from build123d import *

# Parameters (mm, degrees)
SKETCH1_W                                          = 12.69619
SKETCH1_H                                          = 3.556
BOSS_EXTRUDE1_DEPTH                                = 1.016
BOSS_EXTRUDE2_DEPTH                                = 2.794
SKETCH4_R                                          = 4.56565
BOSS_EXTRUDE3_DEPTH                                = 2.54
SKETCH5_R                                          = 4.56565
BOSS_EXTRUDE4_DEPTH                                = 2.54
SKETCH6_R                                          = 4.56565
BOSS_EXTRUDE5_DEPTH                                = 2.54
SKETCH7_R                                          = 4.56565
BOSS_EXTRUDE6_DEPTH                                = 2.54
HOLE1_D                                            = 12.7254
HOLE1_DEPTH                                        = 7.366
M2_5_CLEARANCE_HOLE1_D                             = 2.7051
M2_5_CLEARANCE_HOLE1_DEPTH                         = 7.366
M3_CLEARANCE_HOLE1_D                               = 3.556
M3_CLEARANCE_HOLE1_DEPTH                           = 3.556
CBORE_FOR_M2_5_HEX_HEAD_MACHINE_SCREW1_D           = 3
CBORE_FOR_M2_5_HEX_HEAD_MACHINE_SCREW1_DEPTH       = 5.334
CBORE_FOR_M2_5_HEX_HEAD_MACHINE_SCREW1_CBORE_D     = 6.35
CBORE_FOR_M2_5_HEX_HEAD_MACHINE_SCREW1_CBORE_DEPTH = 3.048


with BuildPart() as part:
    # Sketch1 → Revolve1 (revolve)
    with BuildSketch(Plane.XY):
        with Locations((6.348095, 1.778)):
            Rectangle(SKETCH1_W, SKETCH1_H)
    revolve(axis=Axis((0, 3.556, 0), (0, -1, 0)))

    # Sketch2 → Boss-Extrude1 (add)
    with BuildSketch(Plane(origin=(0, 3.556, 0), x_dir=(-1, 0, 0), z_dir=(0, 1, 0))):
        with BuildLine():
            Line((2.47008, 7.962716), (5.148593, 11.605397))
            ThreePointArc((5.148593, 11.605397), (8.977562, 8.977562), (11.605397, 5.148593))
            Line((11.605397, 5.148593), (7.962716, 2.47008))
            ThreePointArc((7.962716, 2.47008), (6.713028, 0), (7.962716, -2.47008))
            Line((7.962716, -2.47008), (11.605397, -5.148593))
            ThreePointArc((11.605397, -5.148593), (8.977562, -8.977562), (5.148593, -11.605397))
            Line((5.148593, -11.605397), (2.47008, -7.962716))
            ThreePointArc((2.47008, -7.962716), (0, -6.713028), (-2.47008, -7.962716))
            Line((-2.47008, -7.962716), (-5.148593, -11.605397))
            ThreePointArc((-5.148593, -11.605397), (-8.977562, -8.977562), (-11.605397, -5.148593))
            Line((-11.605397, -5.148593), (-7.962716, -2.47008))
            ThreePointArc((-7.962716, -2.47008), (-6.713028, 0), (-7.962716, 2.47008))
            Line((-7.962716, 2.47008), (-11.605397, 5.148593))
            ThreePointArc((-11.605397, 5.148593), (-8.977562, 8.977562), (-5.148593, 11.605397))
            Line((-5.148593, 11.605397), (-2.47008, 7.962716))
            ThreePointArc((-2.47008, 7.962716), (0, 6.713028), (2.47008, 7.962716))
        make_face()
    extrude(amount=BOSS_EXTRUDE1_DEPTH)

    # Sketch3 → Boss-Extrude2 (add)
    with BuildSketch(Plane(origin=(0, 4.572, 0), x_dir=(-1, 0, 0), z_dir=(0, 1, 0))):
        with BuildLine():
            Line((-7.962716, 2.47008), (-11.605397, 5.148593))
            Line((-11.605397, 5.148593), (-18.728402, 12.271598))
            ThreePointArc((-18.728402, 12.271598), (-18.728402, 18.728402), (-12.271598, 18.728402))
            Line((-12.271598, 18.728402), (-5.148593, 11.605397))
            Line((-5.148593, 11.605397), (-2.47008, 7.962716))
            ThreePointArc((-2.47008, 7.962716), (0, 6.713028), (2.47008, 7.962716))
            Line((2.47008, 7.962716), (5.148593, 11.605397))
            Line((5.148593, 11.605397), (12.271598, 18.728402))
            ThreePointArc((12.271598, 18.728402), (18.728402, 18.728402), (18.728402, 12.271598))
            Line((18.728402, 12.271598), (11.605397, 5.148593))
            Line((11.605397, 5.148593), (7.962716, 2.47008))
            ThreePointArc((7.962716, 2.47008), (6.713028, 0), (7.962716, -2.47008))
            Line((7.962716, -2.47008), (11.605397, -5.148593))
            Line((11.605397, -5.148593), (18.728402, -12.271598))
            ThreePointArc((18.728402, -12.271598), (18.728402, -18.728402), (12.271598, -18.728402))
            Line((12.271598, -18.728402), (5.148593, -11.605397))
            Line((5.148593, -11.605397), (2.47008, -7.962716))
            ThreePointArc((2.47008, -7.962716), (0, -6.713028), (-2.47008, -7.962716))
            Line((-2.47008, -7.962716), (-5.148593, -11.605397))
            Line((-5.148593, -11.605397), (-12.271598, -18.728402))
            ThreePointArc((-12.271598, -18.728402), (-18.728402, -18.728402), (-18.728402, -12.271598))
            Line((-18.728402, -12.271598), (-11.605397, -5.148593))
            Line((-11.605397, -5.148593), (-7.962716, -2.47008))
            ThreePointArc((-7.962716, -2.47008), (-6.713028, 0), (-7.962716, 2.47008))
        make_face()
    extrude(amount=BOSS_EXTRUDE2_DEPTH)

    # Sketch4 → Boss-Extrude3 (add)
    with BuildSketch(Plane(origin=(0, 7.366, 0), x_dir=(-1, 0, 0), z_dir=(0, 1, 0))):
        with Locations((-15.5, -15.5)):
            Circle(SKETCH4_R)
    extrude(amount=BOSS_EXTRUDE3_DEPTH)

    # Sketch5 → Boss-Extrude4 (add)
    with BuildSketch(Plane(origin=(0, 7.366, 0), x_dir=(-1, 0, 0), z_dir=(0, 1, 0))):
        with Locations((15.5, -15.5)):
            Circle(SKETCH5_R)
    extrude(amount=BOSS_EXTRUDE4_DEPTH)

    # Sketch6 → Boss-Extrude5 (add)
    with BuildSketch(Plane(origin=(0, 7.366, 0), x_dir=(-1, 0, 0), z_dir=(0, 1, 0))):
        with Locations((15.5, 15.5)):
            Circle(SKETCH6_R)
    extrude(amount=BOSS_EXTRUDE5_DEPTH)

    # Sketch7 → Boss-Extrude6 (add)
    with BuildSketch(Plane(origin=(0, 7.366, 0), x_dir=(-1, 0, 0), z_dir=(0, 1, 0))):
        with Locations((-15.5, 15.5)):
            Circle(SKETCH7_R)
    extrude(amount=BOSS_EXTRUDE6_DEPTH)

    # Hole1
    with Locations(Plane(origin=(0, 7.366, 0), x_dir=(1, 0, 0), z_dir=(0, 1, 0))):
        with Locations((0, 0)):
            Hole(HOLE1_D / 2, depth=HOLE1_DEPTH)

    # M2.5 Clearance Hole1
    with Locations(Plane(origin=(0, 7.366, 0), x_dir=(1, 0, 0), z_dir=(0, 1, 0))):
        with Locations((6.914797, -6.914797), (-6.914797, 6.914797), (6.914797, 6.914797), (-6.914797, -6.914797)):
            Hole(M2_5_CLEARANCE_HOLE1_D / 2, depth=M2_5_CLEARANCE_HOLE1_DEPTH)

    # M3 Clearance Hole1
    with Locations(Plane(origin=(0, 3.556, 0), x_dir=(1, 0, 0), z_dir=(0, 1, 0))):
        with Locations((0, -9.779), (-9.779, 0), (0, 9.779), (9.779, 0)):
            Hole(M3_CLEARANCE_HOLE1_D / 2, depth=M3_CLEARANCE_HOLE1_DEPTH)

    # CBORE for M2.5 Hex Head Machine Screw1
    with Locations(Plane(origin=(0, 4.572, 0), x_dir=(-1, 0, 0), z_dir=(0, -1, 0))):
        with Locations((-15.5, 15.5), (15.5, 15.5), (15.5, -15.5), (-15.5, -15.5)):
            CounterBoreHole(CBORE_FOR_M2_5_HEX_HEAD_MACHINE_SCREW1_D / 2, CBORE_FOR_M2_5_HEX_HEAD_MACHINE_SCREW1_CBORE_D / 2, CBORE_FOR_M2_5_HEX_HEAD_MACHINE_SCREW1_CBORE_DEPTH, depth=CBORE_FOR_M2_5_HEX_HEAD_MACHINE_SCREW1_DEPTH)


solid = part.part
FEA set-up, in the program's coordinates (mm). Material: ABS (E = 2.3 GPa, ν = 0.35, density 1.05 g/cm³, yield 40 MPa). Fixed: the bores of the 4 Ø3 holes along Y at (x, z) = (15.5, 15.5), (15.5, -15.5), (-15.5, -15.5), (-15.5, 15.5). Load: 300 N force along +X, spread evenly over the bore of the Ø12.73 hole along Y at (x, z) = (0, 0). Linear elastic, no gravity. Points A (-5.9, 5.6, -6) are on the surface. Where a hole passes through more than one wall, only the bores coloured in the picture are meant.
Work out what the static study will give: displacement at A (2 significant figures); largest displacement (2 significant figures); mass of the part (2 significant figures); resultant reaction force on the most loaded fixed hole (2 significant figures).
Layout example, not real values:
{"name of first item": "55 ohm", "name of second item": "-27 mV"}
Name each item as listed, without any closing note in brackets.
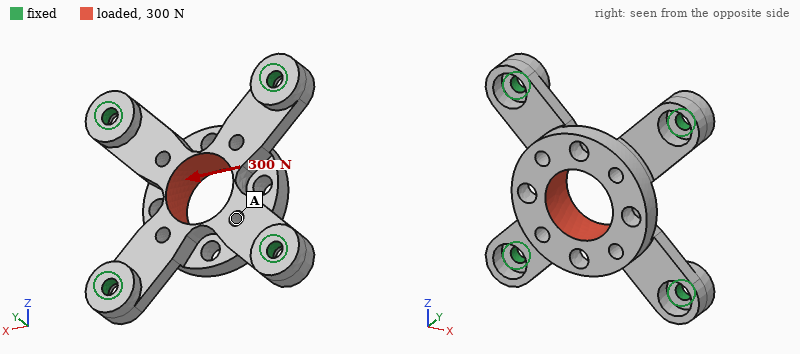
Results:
{"displacement at A": "72 µm", "largest displacement": "98 µm", "mass of the part": "3.6 g", "resultant reaction force on the most loaded fixed hole": "91 N"}
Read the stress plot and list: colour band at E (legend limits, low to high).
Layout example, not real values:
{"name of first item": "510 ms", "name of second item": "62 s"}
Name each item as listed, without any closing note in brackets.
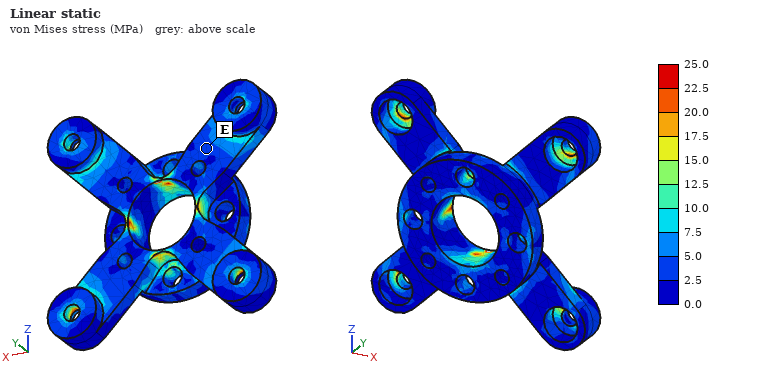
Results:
{"colour band at E": "2.5 to 5.0 MPa"}
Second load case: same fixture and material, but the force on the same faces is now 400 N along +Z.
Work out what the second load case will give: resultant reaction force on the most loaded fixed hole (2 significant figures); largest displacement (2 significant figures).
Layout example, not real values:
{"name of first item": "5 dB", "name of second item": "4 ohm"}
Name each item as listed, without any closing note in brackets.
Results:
{"resultant reaction force on the most loaded fixed hole": "120 N", "largest displacement": "0.13 mm"}
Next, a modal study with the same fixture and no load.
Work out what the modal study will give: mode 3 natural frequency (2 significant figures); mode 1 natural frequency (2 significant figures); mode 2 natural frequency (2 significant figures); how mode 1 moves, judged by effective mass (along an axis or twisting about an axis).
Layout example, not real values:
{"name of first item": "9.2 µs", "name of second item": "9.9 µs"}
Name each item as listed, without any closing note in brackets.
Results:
{"mode 3 natural frequency": "5600 Hz", "mode 1 natural frequency": "4400 Hz", "mode 2 natural frequency": "5600 Hz", "how mode 1 moves, judged by effective mass": "along Y"}
